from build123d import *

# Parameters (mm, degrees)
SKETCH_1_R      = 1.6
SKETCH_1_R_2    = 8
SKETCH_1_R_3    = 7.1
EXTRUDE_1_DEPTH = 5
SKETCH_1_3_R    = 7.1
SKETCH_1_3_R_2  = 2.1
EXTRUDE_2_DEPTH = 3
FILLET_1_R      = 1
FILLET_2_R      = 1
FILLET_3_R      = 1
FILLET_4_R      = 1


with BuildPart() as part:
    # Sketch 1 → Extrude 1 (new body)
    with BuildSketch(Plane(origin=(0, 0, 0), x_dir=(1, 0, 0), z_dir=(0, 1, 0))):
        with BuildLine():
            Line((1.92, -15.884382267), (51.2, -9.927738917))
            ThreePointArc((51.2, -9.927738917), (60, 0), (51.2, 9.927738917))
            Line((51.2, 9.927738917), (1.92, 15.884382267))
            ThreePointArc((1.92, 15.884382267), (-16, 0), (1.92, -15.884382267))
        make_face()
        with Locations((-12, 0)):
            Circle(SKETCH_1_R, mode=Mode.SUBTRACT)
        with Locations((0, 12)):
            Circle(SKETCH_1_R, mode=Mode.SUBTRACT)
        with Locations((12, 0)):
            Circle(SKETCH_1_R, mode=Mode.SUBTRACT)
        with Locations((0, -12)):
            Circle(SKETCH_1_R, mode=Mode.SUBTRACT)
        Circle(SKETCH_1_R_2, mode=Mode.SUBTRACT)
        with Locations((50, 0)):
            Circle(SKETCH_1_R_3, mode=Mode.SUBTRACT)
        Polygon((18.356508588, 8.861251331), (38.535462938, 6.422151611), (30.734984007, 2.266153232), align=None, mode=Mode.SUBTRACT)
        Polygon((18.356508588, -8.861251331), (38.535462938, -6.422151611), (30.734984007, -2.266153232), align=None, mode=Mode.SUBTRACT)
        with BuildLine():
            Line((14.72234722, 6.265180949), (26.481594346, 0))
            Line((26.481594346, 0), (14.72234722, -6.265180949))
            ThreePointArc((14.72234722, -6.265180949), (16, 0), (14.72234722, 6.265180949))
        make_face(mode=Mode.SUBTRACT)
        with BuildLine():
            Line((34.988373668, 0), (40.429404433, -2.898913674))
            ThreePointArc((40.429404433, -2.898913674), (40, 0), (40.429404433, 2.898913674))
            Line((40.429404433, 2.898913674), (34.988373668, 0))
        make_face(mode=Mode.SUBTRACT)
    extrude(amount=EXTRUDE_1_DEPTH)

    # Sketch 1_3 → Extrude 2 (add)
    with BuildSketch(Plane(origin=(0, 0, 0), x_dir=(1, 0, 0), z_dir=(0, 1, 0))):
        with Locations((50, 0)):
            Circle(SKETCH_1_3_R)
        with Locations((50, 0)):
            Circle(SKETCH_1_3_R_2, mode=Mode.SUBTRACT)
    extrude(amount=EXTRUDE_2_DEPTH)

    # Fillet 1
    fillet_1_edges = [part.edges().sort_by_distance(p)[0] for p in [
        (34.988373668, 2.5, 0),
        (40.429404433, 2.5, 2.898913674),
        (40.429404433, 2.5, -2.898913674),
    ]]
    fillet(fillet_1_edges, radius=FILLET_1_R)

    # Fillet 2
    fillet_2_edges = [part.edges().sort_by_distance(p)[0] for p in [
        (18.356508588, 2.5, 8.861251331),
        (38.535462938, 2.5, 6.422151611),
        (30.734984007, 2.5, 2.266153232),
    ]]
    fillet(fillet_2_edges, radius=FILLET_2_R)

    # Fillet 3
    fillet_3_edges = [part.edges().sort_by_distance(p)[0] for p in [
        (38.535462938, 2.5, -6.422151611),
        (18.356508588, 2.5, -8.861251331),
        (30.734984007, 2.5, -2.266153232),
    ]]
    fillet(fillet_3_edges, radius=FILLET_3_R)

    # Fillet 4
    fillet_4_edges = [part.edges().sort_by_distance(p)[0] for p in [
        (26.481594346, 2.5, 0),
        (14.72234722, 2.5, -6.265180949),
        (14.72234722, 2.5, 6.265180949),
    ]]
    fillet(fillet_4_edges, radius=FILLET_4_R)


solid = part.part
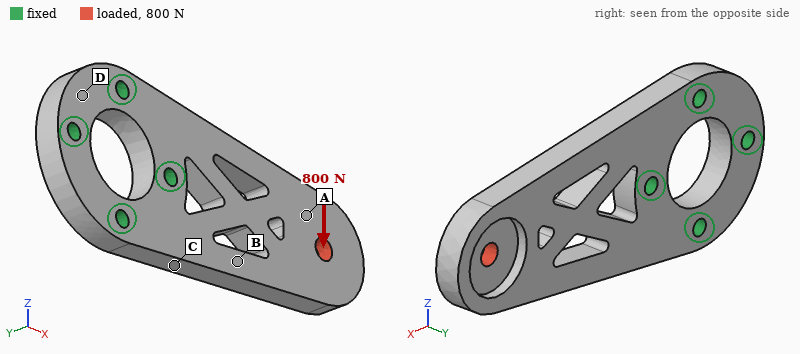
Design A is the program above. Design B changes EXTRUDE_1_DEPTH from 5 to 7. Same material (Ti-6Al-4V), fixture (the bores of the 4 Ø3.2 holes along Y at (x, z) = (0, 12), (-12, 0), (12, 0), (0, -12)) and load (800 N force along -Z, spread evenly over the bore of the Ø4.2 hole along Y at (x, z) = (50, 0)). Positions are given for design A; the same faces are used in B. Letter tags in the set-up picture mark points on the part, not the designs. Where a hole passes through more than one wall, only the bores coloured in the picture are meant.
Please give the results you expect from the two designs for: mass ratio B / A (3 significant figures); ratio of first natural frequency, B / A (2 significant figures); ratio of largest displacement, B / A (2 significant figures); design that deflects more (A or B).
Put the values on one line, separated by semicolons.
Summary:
1.38; 1.4; 0.74; A
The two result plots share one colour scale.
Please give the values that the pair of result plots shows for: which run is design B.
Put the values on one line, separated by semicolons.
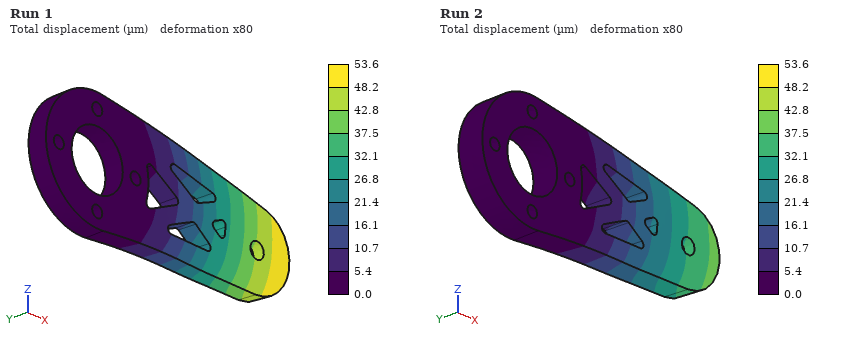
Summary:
Run 2
